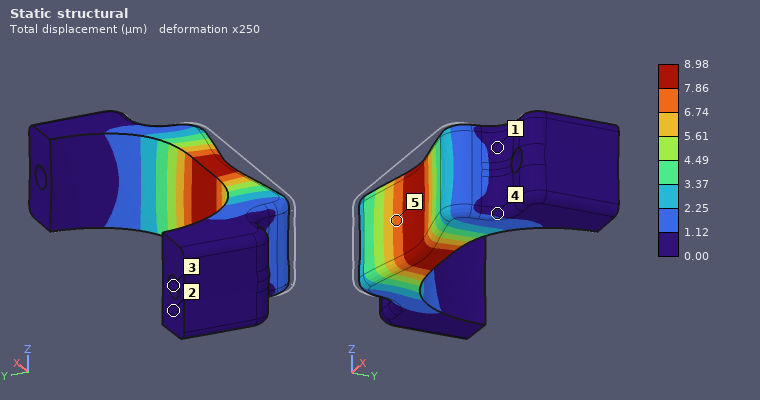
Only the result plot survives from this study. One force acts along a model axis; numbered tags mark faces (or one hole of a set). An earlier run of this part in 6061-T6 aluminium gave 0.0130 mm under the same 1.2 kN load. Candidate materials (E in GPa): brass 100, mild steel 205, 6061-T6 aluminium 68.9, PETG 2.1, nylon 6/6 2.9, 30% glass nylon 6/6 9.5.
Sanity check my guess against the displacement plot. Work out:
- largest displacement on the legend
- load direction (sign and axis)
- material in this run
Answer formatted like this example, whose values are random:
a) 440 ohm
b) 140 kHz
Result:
a) 8.98 µm
b) +Y
c) brass
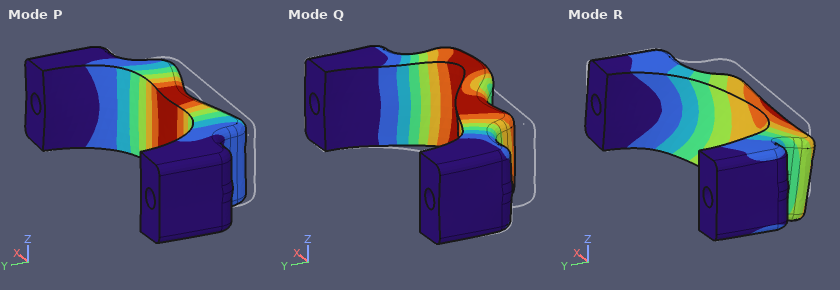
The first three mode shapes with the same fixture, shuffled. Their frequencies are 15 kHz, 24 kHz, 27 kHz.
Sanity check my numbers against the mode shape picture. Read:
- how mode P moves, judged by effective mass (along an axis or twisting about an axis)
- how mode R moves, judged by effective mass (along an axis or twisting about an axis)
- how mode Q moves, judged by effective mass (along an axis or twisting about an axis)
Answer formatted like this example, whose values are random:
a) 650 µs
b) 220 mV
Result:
a) along Y
b) along Z
c) along X
